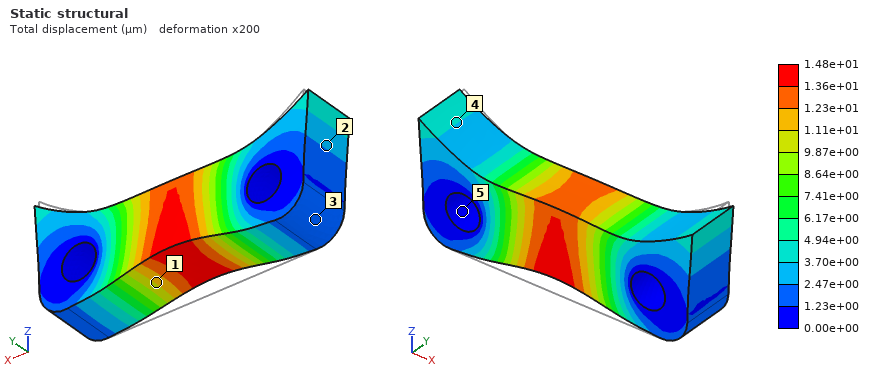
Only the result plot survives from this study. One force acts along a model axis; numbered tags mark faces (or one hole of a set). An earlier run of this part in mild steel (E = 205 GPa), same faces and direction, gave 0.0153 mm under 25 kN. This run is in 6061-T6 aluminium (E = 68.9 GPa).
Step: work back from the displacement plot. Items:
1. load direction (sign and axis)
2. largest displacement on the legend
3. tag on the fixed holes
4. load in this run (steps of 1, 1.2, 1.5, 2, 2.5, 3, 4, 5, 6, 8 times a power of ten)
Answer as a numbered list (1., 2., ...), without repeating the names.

1. +Z
2. 1.48e+01 µm
3. 5
4. 8 kN
